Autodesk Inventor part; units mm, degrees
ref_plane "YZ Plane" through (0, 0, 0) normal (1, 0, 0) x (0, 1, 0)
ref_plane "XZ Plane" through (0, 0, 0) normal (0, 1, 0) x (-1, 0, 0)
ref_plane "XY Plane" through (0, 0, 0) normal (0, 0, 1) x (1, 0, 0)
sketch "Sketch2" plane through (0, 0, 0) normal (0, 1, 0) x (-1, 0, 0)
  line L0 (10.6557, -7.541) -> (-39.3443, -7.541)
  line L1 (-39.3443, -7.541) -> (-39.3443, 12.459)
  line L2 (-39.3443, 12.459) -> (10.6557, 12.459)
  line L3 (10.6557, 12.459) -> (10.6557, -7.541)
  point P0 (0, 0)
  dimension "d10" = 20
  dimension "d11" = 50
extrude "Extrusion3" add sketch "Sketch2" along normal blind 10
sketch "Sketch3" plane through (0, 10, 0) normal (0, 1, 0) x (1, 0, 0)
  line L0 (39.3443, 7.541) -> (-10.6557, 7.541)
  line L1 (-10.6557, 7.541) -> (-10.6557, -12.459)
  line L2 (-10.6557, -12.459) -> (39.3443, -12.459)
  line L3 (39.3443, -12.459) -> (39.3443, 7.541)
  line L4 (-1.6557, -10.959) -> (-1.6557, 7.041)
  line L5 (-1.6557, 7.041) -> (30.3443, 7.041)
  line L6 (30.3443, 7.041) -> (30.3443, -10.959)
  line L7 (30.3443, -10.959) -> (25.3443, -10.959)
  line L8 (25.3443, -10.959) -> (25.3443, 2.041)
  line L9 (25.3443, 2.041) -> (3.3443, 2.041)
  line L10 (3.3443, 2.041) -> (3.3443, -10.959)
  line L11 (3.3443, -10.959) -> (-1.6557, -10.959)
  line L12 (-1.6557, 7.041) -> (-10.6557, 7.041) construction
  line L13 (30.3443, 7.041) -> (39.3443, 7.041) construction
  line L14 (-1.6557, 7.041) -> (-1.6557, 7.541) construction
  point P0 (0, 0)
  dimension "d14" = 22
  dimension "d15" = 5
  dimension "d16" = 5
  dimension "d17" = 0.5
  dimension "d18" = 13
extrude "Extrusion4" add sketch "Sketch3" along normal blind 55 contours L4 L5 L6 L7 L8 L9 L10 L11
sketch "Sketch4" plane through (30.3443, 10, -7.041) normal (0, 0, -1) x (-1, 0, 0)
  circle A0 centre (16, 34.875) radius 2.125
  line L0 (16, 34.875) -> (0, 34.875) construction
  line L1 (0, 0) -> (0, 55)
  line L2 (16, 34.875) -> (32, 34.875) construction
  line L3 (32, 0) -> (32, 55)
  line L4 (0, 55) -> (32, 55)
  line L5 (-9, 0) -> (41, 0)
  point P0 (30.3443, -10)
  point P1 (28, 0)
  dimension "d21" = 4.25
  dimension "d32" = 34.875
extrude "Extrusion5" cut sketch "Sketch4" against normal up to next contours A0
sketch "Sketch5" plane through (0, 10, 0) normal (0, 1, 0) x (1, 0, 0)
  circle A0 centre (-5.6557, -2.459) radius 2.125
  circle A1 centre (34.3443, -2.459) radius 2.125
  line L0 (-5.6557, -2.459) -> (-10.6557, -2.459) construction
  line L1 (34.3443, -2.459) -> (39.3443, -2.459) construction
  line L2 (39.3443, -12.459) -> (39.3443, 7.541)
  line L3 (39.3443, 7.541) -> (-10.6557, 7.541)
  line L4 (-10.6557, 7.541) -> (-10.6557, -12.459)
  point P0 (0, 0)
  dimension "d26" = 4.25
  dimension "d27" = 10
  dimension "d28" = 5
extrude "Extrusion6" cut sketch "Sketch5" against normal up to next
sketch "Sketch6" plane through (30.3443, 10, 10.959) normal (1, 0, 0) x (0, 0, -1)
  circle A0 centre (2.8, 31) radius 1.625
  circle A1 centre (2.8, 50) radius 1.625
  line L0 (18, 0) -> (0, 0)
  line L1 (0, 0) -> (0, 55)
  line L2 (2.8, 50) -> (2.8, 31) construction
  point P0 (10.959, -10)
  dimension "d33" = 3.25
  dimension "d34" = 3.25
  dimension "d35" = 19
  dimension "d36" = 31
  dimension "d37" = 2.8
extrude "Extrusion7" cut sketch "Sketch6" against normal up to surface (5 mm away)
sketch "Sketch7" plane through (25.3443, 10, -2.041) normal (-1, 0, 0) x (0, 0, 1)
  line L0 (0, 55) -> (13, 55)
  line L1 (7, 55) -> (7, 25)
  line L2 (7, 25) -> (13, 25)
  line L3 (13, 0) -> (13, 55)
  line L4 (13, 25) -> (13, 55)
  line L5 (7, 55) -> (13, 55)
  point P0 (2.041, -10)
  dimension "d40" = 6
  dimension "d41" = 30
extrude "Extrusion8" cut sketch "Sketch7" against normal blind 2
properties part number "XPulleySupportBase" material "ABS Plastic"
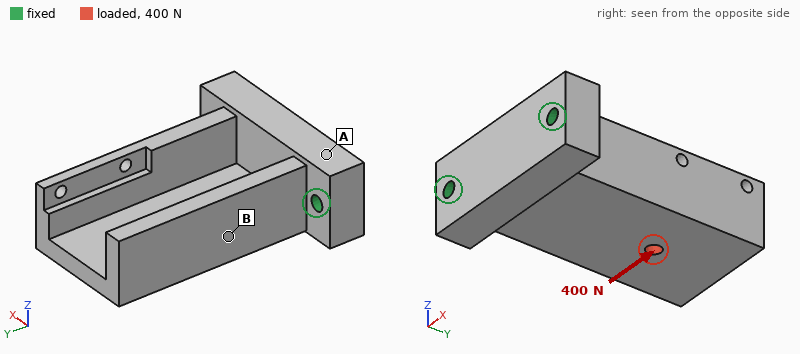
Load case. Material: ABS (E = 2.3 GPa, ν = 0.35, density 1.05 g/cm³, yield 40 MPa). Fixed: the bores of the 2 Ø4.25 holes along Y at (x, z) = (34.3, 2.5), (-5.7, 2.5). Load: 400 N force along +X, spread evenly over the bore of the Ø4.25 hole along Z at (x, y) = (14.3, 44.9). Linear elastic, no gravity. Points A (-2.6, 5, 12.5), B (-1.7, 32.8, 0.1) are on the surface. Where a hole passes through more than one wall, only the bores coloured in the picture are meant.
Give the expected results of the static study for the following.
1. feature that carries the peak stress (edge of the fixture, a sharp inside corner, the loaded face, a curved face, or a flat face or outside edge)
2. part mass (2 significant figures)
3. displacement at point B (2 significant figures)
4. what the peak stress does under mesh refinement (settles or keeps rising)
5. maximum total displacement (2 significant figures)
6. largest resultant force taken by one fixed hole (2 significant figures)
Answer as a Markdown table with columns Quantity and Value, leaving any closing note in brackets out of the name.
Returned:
| Quantity | Value |
|---|---|
| feature that carries the peak stress | edge of the fixture |
| part mass | 26 g |
| displacement at point B | 0.25 mm |
| what the peak stress does under mesh refinement | keeps rising |
| maximum total displacement | 0.71 mm |
| largest resultant force taken by one fixed hole | 480 N |
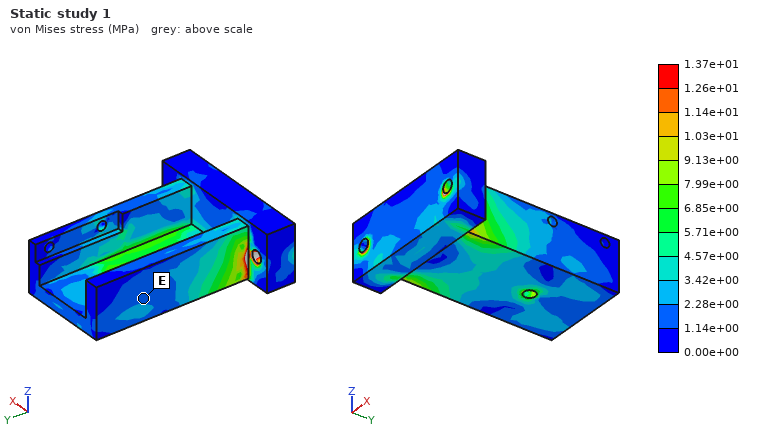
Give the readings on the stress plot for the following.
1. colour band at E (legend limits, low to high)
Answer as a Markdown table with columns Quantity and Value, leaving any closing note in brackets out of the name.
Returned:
| Quantity | Value |
|---|---|
| colour band at E | 1.14e+00 to 2.28e+00 MPa |
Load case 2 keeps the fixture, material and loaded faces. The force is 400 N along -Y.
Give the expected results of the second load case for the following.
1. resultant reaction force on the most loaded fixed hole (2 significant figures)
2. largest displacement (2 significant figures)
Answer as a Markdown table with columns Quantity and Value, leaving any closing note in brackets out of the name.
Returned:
| Quantity | Value |
|---|---|
| resultant reaction force on the most loaded fixed hole | 210 N |
| largest displacement | 0.31 mm |
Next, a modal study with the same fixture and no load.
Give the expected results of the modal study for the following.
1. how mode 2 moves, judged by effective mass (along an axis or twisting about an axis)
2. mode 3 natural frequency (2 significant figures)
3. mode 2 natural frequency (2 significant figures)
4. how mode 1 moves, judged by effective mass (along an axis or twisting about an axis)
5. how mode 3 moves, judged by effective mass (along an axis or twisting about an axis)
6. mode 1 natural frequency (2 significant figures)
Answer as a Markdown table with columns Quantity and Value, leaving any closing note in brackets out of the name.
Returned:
| Quantity | Value |
|---|---|
| how mode 2 moves, judged by effective mass | along X |
| mode 3 natural frequency | 2200 Hz |
| mode 2 natural frequency | 1100 Hz |
| how mode 1 moves, judged by effective mass | along Z |
| how mode 3 moves, judged by effective mass | along X |
| mode 1 natural frequency | 820 Hz |
